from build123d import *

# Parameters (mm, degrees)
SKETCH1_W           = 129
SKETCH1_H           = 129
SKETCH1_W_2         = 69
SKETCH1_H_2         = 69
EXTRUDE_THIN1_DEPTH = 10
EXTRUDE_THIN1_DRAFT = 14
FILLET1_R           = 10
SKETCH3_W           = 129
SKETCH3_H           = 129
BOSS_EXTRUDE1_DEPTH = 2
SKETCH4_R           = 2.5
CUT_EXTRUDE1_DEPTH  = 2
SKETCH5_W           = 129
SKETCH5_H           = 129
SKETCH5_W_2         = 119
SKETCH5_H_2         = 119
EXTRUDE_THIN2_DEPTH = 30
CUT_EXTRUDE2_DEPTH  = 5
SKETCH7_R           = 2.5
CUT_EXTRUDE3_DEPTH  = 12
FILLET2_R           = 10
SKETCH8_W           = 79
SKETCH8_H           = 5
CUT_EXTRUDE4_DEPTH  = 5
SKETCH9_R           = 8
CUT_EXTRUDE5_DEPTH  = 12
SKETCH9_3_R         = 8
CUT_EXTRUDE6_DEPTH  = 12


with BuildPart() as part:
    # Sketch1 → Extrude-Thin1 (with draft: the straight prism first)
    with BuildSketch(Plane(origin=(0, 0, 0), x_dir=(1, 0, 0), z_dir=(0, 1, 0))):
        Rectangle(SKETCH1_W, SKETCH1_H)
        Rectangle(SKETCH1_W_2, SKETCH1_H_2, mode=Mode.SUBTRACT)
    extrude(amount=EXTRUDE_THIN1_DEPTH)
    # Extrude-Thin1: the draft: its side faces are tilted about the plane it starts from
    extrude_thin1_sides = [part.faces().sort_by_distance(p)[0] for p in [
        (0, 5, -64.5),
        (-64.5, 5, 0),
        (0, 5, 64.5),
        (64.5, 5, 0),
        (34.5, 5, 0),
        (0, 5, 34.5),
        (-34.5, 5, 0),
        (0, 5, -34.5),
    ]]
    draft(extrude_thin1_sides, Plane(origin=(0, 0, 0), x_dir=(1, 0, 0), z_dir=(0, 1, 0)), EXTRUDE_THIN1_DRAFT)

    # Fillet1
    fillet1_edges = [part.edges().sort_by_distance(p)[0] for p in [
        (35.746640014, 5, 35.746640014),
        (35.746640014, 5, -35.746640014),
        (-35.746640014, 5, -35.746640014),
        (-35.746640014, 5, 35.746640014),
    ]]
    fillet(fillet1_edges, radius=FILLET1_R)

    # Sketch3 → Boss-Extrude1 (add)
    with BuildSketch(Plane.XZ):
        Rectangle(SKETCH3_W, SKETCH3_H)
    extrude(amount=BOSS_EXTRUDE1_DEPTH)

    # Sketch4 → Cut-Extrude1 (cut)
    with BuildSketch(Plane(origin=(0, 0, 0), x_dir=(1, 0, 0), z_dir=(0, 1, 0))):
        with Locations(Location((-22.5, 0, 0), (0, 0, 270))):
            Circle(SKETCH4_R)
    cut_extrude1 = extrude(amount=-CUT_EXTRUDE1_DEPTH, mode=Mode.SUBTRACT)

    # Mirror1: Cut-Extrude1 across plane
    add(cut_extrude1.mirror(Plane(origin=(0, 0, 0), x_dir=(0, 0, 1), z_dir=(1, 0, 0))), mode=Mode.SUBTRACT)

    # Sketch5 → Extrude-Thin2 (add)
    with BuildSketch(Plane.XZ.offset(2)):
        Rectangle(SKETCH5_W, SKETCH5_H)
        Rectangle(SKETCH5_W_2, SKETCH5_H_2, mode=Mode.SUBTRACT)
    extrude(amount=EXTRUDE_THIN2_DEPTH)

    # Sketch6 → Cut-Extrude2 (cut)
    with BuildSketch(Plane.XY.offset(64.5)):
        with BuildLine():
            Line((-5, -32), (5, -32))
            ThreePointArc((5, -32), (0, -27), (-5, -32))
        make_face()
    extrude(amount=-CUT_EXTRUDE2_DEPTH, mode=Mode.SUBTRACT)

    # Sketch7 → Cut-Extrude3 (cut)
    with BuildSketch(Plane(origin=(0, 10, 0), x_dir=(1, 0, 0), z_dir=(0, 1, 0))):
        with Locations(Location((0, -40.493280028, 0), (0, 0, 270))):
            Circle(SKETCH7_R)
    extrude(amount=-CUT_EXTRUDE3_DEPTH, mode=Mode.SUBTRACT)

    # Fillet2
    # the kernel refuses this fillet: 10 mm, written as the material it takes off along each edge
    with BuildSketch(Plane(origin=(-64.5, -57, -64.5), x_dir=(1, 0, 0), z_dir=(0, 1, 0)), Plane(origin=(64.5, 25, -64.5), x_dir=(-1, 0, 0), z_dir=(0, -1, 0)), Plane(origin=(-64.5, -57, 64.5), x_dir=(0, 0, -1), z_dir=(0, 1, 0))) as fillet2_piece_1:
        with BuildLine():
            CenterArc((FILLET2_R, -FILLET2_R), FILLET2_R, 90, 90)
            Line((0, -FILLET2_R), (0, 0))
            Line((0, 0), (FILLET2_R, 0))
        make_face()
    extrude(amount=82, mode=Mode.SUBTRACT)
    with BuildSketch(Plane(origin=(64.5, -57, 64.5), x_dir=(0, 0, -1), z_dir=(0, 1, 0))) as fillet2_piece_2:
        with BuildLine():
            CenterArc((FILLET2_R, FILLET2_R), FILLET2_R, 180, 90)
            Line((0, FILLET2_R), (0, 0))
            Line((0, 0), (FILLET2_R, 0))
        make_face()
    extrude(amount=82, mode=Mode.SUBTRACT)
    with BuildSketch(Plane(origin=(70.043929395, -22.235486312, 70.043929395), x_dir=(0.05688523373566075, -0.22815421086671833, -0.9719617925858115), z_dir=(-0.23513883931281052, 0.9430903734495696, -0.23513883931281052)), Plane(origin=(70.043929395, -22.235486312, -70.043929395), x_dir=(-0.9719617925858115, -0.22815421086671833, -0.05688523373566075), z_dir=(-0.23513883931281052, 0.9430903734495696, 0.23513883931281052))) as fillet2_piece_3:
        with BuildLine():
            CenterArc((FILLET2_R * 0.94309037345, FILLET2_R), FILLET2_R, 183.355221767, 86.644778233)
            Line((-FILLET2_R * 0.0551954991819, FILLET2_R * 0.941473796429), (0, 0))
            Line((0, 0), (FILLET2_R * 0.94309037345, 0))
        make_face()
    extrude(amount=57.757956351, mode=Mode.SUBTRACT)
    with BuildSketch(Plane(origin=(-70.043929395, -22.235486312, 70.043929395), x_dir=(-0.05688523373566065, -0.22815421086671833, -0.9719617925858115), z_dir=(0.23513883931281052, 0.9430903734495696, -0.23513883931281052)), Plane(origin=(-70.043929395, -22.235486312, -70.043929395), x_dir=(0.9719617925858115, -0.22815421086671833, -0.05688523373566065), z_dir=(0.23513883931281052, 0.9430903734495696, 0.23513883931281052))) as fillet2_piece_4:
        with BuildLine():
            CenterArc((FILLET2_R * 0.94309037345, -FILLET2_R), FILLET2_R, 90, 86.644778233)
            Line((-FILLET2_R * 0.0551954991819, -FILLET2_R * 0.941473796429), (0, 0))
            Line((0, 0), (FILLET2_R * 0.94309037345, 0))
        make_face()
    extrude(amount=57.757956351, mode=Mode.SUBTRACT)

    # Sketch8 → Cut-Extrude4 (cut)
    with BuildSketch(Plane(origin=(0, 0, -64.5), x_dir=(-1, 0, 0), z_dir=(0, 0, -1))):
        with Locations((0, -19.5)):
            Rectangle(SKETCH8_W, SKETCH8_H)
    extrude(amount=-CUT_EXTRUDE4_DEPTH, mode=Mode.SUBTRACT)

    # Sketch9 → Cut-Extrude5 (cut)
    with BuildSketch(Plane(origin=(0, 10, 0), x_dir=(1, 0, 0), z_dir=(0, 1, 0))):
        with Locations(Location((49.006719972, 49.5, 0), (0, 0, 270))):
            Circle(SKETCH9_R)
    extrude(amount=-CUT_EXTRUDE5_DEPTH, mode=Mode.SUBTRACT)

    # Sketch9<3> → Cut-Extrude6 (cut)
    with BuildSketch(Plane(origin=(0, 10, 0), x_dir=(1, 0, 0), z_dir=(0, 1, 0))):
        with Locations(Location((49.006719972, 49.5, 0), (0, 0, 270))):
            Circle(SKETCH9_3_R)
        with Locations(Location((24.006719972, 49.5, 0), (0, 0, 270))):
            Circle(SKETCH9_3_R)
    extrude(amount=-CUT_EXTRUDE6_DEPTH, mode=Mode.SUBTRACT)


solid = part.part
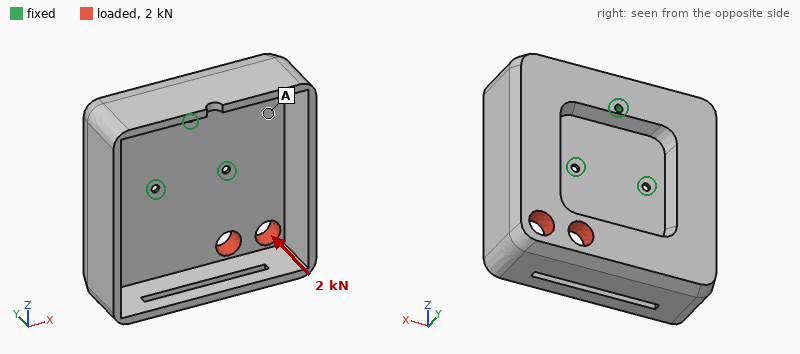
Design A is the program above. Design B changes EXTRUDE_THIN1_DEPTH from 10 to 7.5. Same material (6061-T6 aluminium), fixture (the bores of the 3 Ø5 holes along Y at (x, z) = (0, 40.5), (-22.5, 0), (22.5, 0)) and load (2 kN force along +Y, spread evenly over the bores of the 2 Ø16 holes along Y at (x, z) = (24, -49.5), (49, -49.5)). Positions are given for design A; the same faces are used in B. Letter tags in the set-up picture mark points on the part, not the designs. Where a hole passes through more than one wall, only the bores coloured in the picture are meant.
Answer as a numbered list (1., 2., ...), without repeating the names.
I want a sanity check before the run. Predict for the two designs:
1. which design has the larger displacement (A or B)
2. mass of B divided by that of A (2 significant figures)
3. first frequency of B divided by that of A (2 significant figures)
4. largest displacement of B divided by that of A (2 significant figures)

1. B
2. 0.88
3. 0.93
4. 1.4
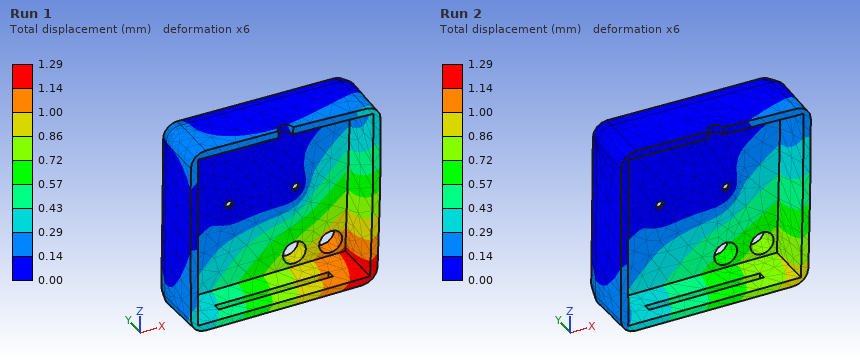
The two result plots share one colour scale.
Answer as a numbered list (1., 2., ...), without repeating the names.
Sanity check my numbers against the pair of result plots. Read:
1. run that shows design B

1. Run 1
